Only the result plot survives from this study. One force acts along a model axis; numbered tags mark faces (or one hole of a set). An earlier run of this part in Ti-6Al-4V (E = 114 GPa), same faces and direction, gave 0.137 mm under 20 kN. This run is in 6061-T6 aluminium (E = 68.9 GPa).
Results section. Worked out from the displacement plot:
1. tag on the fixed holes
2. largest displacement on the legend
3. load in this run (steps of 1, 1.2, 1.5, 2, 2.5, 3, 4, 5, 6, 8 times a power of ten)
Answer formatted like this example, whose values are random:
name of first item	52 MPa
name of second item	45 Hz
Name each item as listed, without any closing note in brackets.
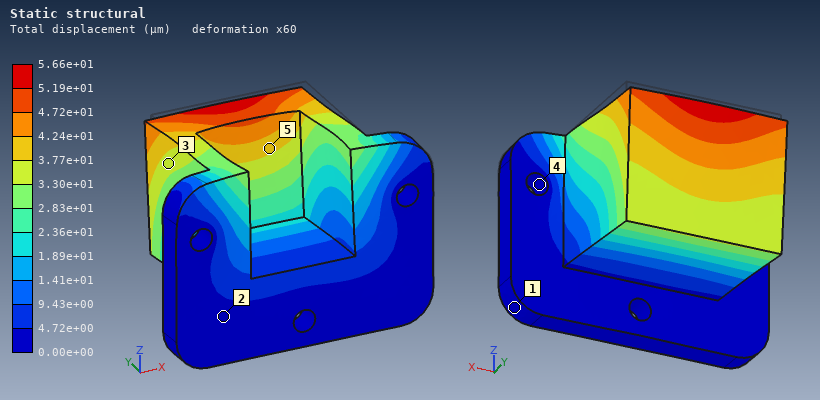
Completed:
tag on the fixed holes	4
largest displacement on the legend	5.66e+01 µm
load in this run	5 kN
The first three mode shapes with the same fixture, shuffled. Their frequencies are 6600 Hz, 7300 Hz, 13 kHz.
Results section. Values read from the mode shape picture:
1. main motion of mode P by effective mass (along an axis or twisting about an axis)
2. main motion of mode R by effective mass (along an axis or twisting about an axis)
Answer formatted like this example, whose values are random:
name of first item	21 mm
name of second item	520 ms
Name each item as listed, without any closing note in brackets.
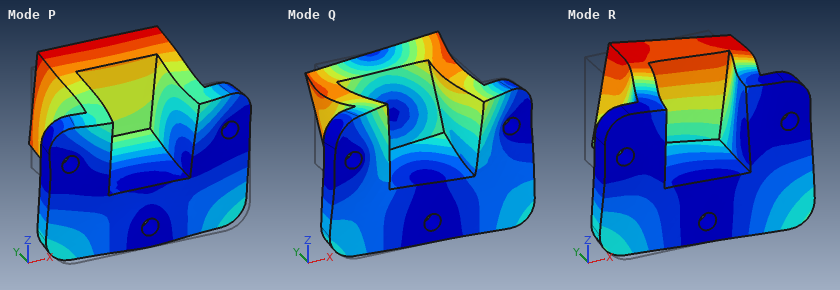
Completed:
main motion of mode P by effective mass	along Z
main motion of mode R by effective mass	along X
